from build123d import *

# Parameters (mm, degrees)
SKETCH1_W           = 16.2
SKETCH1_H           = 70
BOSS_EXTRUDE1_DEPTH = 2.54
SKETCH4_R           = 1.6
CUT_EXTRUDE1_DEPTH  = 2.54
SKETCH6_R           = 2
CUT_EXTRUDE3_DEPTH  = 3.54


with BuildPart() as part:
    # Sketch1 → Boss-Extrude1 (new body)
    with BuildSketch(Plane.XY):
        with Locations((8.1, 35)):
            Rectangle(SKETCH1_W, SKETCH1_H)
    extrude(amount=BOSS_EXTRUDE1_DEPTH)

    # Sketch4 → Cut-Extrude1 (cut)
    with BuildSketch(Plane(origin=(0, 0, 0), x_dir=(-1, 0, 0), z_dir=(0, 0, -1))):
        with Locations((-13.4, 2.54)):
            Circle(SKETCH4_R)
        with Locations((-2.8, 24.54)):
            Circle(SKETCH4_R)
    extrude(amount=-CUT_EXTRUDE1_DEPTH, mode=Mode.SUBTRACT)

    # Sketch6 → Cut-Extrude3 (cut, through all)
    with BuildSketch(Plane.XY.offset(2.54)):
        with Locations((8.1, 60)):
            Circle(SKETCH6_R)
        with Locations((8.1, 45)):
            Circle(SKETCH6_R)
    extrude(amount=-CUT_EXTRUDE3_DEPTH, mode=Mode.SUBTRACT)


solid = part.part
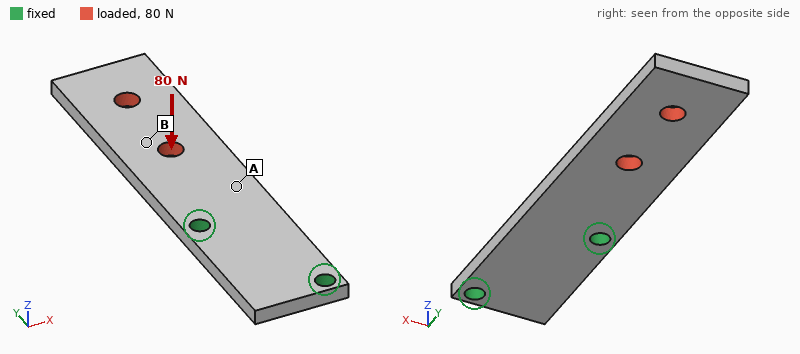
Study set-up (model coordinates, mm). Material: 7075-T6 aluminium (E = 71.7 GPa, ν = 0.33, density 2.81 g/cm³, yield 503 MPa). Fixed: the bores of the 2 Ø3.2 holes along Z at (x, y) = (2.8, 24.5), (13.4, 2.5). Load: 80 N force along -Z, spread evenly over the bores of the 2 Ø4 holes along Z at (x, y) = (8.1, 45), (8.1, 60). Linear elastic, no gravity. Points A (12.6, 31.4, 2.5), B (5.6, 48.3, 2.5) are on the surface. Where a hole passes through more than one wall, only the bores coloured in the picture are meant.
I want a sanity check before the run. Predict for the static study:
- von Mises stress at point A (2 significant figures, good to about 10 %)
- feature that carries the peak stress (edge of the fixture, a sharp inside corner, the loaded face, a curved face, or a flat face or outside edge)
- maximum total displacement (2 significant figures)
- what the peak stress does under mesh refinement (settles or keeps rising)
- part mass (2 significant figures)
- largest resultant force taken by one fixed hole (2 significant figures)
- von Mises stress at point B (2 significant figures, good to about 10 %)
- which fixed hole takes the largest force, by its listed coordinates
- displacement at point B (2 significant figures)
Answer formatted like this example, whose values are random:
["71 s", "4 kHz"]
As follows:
["83 MPa", "edge of the fixture", "0.81 mm", "keeps rising", "7.8 g", "110 N", "29 MPa", "(2.8, 24.5)", "0.31 mm"]
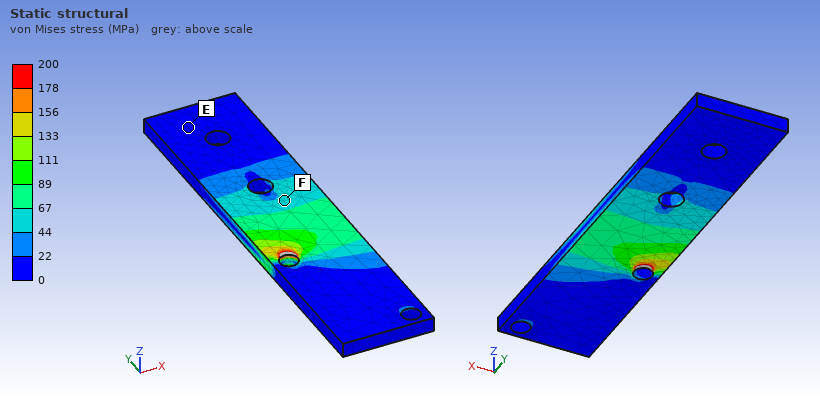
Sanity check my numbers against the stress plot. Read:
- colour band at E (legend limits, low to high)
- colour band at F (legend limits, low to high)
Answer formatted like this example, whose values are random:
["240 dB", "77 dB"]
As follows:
["0 to 22 MPa", "44 to 67 MPa"]
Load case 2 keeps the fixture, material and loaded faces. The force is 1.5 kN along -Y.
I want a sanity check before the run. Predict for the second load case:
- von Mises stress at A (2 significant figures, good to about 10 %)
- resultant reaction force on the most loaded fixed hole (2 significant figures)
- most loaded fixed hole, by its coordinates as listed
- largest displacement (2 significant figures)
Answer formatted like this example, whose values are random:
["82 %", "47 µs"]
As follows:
["36 MPa", "1.1 kN", "(2.8, 24.5)", "45 µm"]
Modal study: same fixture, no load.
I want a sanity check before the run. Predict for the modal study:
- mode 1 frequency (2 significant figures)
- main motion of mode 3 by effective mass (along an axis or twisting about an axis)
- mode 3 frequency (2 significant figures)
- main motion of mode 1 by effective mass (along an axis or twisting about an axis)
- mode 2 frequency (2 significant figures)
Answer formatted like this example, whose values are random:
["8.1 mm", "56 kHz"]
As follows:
["990 Hz", "along X", "4900 Hz", "along Z", "4600 Hz"]
